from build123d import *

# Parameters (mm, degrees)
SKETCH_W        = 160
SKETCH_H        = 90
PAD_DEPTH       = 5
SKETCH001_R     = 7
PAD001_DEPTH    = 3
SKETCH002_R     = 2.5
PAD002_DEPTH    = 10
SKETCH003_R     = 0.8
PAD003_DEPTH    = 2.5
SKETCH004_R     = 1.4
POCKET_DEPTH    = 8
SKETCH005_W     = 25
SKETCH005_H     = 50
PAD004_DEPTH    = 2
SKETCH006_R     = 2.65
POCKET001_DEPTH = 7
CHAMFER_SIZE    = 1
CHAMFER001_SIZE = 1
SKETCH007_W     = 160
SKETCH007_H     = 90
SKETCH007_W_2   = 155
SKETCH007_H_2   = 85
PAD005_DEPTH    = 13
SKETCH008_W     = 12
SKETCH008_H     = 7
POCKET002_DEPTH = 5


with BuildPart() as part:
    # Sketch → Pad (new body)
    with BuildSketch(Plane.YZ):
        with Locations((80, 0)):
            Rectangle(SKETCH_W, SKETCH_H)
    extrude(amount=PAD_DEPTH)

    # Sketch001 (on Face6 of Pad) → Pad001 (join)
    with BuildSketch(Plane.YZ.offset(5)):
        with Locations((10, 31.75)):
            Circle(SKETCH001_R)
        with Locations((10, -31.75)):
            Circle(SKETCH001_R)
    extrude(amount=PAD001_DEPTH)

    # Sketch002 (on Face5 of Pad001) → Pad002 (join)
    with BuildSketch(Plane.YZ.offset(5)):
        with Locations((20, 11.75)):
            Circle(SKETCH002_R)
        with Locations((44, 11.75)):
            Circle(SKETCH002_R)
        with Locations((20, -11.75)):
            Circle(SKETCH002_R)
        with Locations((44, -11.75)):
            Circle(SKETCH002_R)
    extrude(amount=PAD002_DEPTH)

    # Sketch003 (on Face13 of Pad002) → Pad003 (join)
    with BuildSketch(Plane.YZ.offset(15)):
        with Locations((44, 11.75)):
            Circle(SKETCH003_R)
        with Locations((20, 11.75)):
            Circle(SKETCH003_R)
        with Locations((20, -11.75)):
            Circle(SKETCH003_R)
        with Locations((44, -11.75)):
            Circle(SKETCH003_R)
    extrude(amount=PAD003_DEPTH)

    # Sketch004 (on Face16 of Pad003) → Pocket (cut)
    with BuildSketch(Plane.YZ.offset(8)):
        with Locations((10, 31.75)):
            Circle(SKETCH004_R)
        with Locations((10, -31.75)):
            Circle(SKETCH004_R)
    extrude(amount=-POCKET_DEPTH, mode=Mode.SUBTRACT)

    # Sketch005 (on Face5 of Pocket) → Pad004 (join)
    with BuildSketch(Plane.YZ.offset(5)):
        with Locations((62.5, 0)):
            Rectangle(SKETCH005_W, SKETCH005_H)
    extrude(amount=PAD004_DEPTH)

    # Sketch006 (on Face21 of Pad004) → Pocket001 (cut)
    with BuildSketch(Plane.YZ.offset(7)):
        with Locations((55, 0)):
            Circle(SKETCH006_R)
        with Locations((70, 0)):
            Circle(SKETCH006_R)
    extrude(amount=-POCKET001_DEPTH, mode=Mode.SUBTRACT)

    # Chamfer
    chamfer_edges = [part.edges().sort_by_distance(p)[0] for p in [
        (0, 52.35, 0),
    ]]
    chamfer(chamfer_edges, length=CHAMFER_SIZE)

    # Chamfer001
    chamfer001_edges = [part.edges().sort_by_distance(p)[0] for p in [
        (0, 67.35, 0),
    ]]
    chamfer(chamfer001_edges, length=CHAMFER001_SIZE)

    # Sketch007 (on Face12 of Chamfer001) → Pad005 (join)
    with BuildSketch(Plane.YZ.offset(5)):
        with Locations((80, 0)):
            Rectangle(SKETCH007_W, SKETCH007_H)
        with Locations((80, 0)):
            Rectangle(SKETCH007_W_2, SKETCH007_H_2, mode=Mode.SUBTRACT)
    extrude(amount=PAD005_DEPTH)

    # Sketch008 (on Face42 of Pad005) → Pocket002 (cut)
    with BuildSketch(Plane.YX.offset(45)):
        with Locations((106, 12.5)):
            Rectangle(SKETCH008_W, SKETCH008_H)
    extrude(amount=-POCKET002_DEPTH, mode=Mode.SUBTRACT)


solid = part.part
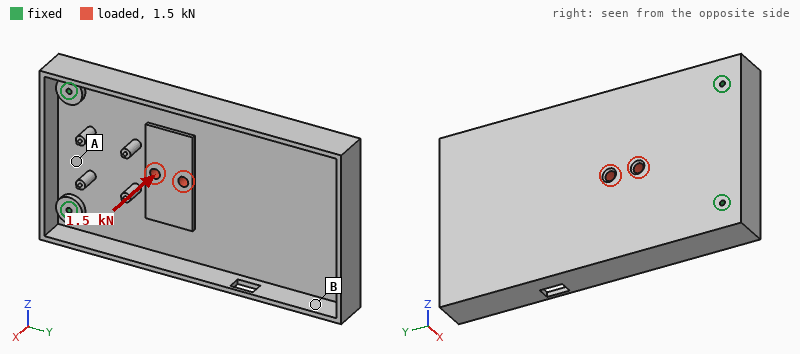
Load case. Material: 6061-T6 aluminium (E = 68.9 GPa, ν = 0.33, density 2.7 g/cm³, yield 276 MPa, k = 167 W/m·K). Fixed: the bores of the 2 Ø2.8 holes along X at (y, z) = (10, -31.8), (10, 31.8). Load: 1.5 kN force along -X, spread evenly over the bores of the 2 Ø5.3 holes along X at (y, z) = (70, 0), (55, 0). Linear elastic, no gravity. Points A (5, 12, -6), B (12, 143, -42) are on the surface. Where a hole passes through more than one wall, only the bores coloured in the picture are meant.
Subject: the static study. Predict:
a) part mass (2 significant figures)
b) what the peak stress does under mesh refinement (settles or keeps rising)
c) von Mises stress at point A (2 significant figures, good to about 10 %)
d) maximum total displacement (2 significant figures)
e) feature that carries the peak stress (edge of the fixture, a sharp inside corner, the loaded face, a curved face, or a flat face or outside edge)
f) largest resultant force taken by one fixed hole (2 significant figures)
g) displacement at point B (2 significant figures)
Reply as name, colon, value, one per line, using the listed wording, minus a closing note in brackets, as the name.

part mass: 250 g
what the peak stress does under mesh refinement: keeps rising
von Mises stress at point A: 42 MPa
maximum total displacement: 1.7 mm
feature that carries the peak stress: edge of the fixture
largest resultant force taken by one fixed hole: 900 N
displacement at point B: 1.5 mm
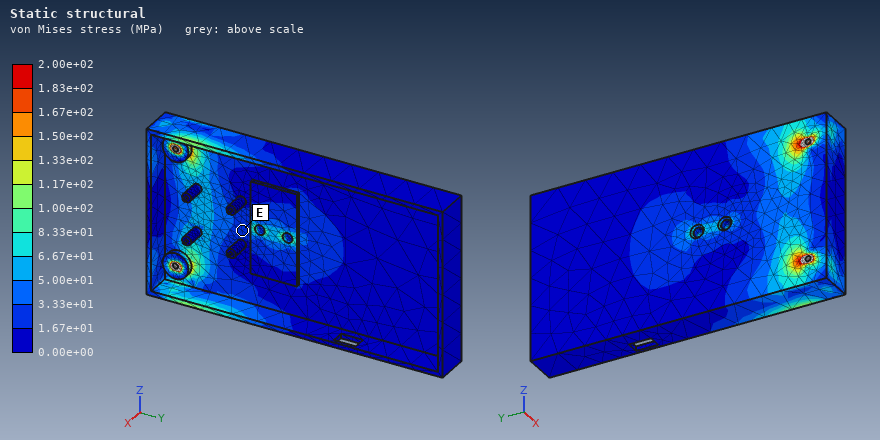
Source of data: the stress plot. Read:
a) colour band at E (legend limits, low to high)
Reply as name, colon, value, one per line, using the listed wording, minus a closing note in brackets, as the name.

colour band at E: 1.67e+01 to 3.33e+01 MPa
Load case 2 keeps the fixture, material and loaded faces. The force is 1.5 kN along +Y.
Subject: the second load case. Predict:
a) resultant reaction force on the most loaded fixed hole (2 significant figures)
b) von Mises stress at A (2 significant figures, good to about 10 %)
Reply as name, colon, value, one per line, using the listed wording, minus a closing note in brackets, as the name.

resultant reaction force on the most loaded fixed hole: 760 N
von Mises stress at A: 1.7 MPa
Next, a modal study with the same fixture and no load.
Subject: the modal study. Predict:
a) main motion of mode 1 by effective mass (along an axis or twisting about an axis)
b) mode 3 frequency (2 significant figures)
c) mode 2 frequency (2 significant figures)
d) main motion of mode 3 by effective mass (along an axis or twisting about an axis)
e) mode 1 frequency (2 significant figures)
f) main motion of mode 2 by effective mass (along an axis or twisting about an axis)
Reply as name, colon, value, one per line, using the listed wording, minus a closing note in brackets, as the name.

main motion of mode 1 by effective mass: along X
mode 3 frequency: 1800 Hz
mode 2 frequency: 670 Hz
main motion of mode 3 by effective mass: along X
mode 1 frequency: 280 Hz
main motion of mode 2 by effective mass: twisting about Y
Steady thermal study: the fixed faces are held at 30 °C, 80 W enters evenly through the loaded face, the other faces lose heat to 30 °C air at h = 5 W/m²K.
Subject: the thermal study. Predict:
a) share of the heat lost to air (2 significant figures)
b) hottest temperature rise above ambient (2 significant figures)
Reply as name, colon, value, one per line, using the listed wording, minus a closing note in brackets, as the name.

share of the heat lost to air: 11 %
hottest temperature rise above ambient: 68 K
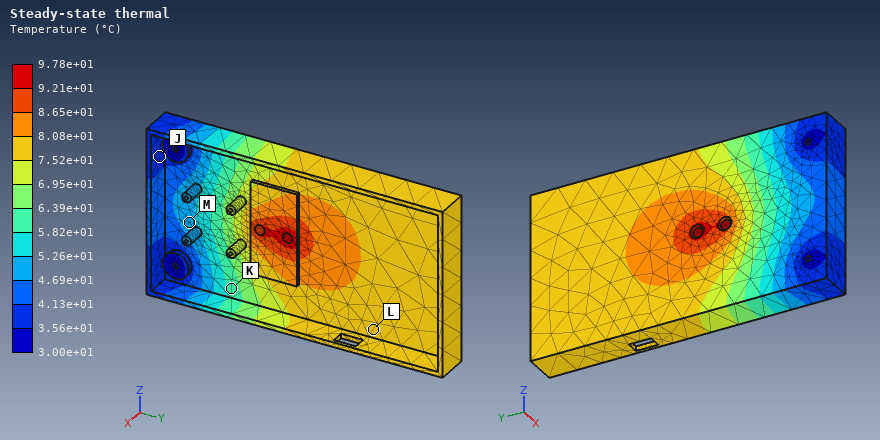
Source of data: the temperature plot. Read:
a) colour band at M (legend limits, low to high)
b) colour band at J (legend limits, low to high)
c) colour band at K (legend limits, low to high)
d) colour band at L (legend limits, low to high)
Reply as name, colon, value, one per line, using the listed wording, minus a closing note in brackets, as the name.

colour band at M: 4.69e+01 to 5.26e+01 °C
colour band at J: 3.56e+01 to 4.13e+01 °C
colour band at K: 5.82e+01 to 6.39e+01 °C
colour band at L: 7.52e+01 to 8.08e+01 °C
